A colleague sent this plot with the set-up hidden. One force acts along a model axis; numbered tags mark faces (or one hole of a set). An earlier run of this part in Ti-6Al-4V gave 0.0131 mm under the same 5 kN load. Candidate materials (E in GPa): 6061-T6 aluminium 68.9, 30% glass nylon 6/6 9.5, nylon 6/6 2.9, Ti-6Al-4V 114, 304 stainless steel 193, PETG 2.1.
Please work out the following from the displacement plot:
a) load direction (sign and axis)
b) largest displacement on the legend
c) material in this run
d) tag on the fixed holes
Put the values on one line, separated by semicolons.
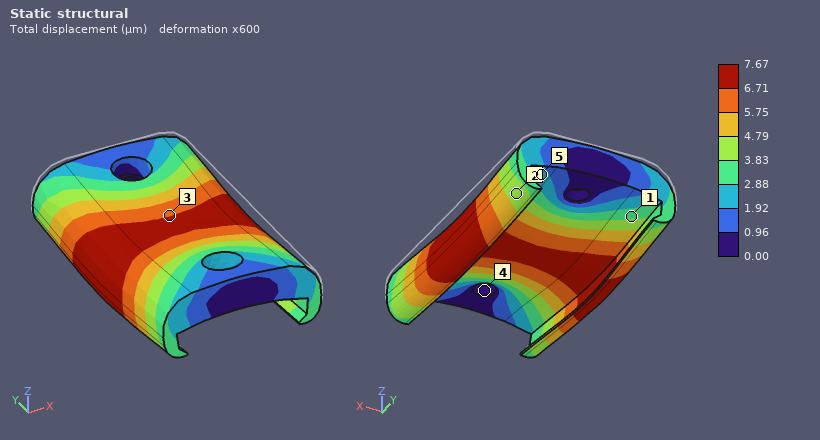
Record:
-Z; 7.67 µm; 304 stainless steel; 4
